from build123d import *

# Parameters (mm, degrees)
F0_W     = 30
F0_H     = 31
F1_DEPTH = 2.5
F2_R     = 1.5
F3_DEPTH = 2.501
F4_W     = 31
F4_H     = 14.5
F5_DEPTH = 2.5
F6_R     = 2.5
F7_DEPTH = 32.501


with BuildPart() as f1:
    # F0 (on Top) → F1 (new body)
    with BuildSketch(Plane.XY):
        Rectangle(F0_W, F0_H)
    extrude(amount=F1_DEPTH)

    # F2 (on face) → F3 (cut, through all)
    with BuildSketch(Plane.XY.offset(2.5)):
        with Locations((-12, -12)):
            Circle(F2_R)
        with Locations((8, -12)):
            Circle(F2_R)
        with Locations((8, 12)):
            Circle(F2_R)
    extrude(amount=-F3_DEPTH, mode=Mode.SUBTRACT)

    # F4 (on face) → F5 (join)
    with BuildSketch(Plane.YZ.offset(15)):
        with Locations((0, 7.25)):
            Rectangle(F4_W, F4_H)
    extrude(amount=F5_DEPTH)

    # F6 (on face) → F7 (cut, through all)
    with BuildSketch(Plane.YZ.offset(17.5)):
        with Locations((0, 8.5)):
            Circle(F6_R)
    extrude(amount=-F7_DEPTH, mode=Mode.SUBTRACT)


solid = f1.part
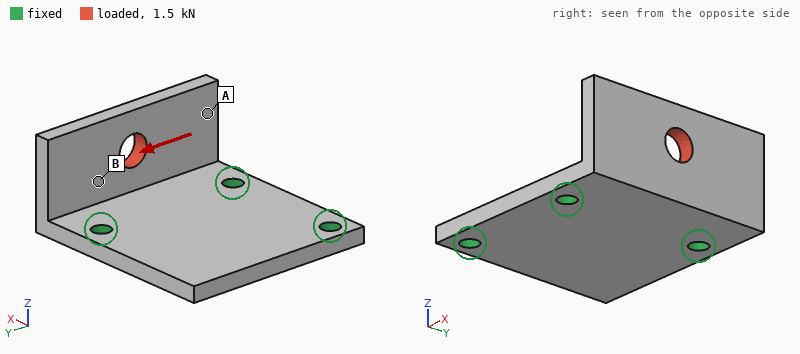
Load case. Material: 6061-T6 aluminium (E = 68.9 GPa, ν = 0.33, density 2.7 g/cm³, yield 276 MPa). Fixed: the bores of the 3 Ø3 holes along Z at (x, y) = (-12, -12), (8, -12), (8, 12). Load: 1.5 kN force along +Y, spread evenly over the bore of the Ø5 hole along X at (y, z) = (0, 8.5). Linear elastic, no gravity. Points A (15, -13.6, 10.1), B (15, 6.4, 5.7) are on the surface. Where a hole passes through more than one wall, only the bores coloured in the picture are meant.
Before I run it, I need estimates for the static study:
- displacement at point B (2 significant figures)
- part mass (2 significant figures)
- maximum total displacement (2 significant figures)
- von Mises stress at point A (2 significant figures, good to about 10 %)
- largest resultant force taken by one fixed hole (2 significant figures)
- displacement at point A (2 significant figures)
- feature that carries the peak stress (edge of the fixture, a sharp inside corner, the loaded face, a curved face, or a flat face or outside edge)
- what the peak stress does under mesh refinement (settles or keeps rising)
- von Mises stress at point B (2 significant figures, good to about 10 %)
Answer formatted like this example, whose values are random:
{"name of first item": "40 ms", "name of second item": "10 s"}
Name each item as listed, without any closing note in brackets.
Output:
{"displacement at point B": "0.037 mm", "part mass": "9.0 g", "maximum total displacement": "0.11 mm", "von Mises stress at point A": "29 MPa", "largest resultant force taken by one fixed hole": "990 N", "displacement at point A": "0.080 mm", "feature that carries the peak stress": "edge of the fixture", "what the peak stress does under mesh refinement": "keeps rising", "von Mises stress at point B": "78 MPa"}
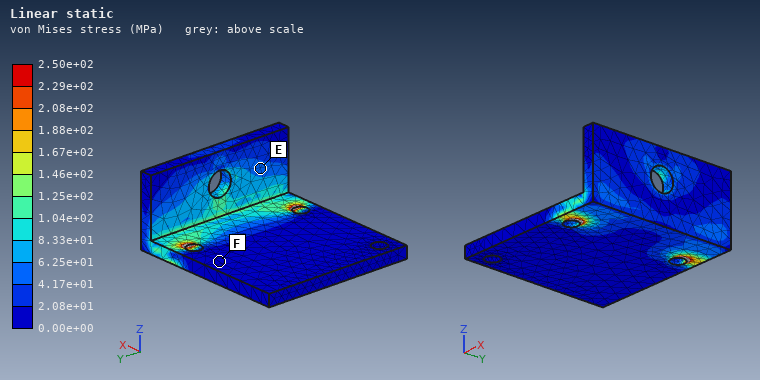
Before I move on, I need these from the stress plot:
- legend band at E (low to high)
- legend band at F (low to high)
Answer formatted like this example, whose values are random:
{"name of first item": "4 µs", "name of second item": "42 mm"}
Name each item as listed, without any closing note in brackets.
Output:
{"legend band at E": "4.17e+01 to 6.25e+01 MPa", "legend band at F": "0.00e+00 to 2.08e+01 MPa"}
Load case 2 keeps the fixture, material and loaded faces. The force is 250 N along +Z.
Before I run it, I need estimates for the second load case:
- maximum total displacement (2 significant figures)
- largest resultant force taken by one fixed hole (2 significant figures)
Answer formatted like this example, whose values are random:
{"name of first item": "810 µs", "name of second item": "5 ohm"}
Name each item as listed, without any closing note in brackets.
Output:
{"maximum total displacement": "48 µm", "largest resultant force taken by one fixed hole": "140 N"}
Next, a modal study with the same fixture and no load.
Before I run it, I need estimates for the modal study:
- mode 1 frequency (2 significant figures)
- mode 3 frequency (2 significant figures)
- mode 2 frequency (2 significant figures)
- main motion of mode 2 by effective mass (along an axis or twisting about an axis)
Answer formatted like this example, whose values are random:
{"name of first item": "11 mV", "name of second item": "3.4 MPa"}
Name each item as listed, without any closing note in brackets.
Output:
{"mode 1 frequency": "5800 Hz", "mode 3 frequency": "10 kHz", "mode 2 frequency": "6700 Hz", "main motion of mode 2 by effective mass": "along Z"}
